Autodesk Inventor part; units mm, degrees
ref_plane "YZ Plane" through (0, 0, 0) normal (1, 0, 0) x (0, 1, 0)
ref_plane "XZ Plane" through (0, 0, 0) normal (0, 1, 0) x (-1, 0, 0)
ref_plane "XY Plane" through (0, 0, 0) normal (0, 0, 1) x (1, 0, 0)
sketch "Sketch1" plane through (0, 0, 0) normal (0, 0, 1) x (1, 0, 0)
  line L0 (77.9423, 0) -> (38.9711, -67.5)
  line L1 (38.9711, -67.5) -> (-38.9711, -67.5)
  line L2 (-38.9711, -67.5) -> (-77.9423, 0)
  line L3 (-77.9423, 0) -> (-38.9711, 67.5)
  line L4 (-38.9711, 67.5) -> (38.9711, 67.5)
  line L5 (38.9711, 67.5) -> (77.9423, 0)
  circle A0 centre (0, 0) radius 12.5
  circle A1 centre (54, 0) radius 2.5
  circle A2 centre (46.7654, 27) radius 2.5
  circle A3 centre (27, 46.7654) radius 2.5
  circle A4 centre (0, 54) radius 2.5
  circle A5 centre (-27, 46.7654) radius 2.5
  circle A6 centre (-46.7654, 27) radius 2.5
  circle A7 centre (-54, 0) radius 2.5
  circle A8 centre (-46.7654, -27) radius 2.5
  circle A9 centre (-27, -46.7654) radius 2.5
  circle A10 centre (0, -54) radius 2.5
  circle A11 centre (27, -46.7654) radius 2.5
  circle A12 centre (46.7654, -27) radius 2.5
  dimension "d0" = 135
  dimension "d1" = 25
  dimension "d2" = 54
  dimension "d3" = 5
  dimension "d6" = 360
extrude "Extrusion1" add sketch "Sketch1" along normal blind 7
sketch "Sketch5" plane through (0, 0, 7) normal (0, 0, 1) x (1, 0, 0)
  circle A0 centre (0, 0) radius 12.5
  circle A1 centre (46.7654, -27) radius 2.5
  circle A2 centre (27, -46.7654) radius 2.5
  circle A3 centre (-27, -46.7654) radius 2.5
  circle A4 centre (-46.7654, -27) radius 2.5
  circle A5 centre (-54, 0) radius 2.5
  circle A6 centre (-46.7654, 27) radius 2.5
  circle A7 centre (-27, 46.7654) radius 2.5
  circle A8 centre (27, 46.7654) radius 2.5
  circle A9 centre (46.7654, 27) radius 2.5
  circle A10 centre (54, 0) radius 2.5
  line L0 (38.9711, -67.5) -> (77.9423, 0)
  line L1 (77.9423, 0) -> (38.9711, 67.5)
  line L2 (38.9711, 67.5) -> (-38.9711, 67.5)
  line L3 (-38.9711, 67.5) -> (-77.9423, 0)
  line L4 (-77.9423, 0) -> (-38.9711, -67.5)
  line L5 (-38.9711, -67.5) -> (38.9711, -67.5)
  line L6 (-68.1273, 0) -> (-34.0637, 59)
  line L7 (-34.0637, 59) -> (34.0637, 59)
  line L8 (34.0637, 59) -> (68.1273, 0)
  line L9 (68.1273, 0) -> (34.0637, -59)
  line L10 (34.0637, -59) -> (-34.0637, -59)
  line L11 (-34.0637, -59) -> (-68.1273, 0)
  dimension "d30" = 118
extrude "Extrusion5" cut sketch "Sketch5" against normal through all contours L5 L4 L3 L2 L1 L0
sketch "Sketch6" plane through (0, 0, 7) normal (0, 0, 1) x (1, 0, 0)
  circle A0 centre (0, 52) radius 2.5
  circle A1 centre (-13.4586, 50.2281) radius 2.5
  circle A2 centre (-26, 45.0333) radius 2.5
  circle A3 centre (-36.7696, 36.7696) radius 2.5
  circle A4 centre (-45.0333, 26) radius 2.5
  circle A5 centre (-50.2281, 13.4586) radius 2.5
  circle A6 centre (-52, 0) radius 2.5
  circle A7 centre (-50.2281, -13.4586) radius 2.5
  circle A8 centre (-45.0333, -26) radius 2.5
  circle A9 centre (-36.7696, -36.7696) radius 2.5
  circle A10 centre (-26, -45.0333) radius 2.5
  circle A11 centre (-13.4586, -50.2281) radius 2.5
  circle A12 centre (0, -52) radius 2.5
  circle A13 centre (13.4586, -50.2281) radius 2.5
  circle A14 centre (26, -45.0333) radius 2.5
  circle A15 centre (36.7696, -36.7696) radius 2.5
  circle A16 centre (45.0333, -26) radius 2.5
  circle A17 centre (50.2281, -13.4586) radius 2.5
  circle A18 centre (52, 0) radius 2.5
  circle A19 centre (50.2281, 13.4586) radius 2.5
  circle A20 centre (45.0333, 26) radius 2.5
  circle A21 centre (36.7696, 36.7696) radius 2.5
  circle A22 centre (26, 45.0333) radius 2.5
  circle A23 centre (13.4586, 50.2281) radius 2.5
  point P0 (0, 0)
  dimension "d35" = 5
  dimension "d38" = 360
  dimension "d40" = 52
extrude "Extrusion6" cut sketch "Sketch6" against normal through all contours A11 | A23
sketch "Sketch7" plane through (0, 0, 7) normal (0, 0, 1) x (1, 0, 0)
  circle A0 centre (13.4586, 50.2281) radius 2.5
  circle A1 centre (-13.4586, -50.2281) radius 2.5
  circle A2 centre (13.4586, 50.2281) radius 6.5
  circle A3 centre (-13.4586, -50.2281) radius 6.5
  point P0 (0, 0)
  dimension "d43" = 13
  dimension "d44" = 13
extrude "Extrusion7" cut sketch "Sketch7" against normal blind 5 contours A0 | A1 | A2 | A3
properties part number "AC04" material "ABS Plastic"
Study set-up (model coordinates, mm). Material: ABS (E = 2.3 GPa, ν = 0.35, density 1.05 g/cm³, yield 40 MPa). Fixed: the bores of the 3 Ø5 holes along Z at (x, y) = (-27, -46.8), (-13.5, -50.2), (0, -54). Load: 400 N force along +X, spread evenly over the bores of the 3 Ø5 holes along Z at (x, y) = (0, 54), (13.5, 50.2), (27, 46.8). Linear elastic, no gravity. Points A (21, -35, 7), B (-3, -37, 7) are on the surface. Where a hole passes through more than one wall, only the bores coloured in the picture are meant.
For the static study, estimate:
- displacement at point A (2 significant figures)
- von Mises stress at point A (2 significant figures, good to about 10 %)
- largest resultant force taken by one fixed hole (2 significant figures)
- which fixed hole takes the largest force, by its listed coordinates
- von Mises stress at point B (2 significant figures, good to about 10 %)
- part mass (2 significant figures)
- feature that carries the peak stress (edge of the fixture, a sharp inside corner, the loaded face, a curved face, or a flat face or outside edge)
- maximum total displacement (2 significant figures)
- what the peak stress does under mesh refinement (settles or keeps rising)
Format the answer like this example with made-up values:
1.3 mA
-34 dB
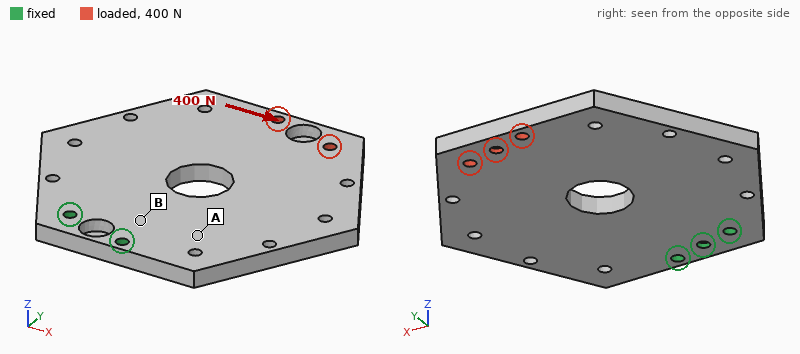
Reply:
0.26 mm
2.7 MPa
1.3 kN
(-27, -46.8)
7.3 MPa
82 g
edge of the fixture
0.99 mm
keeps rising
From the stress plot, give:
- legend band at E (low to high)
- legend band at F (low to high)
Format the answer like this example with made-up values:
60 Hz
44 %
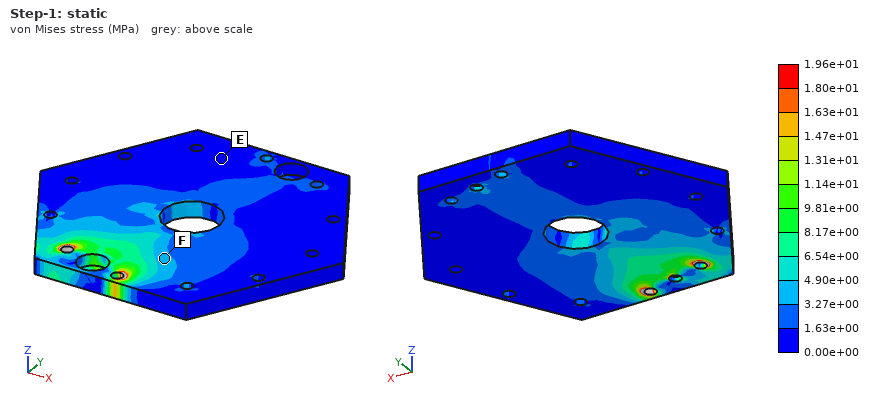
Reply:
0.00e+00 to 1.63e+00 MPa
3.27e+00 to 4.90e+00 MPa
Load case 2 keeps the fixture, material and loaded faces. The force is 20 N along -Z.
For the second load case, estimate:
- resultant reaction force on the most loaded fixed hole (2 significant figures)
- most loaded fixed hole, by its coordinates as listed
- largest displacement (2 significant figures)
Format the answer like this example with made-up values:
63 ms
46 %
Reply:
76 N
(-13.5, -50.2)
1.8 mm
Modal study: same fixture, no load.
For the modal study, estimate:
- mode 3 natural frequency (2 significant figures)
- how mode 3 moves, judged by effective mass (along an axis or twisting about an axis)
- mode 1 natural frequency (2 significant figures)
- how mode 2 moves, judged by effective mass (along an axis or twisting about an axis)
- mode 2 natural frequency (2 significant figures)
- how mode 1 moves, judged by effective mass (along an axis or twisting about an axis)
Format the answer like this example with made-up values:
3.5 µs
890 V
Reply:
580 Hz
along X
120 Hz
twisting about Y
260 Hz
along Z
